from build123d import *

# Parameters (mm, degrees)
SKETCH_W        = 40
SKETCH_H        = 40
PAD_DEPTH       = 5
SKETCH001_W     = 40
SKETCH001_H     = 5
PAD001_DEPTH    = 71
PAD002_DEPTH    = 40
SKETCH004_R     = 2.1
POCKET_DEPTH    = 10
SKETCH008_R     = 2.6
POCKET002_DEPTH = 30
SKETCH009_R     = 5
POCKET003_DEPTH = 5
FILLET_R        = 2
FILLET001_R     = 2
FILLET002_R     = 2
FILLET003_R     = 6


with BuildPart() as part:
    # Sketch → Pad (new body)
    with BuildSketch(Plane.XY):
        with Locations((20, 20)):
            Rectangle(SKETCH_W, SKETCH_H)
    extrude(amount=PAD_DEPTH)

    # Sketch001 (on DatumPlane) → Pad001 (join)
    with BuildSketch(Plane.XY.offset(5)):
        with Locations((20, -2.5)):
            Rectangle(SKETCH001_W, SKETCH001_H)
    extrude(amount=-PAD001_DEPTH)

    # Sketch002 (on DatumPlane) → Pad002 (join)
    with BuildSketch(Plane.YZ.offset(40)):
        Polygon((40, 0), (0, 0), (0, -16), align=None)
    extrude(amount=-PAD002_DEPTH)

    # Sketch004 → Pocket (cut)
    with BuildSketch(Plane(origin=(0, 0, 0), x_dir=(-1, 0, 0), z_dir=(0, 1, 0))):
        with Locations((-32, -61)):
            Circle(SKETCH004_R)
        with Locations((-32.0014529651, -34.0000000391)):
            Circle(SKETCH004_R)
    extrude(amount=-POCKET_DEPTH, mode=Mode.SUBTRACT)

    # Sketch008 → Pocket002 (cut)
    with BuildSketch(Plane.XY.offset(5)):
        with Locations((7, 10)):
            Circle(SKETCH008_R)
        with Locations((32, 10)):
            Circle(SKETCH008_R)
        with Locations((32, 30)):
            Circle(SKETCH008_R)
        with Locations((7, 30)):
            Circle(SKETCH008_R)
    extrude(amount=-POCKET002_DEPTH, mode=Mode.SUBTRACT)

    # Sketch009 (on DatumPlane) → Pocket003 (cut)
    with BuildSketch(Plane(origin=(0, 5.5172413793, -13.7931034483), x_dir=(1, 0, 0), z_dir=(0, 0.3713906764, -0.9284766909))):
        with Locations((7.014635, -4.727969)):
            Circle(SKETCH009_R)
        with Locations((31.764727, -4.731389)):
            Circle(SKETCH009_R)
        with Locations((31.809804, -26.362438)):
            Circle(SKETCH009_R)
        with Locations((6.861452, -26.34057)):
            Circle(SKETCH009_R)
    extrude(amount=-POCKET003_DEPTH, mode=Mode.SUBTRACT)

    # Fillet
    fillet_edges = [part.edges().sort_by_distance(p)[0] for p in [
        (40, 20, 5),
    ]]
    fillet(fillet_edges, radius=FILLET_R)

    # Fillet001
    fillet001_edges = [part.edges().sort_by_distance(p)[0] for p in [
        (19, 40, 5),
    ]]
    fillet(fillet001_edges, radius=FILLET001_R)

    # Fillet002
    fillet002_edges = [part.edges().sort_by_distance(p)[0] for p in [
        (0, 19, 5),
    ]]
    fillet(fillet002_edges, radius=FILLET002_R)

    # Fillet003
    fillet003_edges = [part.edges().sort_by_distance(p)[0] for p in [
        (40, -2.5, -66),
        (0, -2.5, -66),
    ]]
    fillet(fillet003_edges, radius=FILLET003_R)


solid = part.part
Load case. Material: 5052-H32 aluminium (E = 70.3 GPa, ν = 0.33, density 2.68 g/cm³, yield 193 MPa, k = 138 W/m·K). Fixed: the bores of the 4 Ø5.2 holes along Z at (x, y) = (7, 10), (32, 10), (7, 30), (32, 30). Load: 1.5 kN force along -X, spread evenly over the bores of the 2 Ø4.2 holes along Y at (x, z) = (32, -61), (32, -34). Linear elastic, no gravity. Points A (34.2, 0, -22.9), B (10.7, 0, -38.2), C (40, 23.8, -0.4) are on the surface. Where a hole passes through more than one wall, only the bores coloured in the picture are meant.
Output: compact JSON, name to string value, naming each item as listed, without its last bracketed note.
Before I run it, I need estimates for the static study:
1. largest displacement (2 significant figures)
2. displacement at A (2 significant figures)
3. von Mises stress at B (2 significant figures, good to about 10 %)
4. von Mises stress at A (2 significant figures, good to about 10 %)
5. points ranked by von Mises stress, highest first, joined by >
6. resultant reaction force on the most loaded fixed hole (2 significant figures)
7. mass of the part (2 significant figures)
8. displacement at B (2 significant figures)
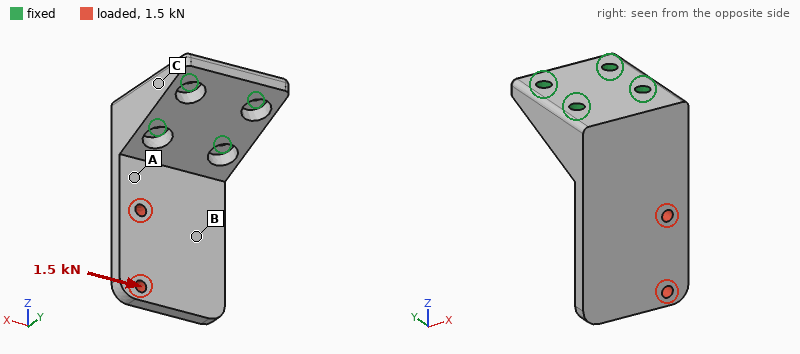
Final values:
{"largest displacement": "75 µm", "displacement at A": "21 µm", "von Mises stress at B": "13 MPa", "von Mises stress at A": "28 MPa", "points ranked by von Mises stress, highest first, joined by >": "A > B > C", "resultant reaction force on the most loaded fixed hole": "2.4 kN", "mass of the part": "87 g", "displacement at B": "36 µm"}
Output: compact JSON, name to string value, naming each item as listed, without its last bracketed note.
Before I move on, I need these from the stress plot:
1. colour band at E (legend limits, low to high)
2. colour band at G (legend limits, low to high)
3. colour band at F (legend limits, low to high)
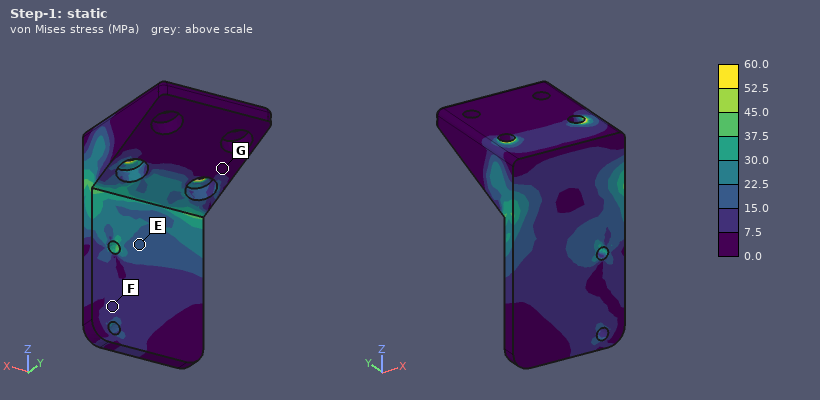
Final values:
{"colour band at E": "15.0 to 22.5 MPa", "colour band at G": "0.0 to 7.5 MPa", "colour band at F": "7.5 to 15.0 MPa"}
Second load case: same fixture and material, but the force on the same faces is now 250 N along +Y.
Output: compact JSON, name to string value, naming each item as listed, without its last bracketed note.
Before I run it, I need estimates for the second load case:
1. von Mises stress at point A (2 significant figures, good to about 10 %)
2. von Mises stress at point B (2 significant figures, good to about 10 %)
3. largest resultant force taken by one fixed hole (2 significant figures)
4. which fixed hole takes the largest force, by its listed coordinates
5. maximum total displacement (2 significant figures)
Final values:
{"von Mises stress at point A": "39 MPa", "von Mises stress at point B": "20 MPa", "largest resultant force taken by one fixed hole": "220 N", "which fixed hole takes the largest force, by its listed coordinates": "(32, 10)", "maximum total displacement": "0.26 mm"}
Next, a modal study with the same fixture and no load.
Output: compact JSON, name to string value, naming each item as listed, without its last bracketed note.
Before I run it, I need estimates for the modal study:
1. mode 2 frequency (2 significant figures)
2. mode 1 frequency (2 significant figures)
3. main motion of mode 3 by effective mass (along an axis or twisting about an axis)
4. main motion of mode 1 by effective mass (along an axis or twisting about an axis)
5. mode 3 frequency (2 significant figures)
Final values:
{"mode 2 frequency": "4300 Hz", "mode 1 frequency": "1500 Hz", "main motion of mode 3 by effective mass": "along X", "main motion of mode 1 by effective mass": "along Y", "mode 3 frequency": "6000 Hz"}
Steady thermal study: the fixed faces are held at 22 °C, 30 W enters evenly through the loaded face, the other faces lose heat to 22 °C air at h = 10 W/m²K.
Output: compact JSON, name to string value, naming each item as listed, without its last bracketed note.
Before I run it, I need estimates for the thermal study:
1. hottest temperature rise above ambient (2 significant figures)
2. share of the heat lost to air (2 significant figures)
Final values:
{"hottest temperature rise above ambient": "55 K", "share of the heat lost to air": "5.1 %"}
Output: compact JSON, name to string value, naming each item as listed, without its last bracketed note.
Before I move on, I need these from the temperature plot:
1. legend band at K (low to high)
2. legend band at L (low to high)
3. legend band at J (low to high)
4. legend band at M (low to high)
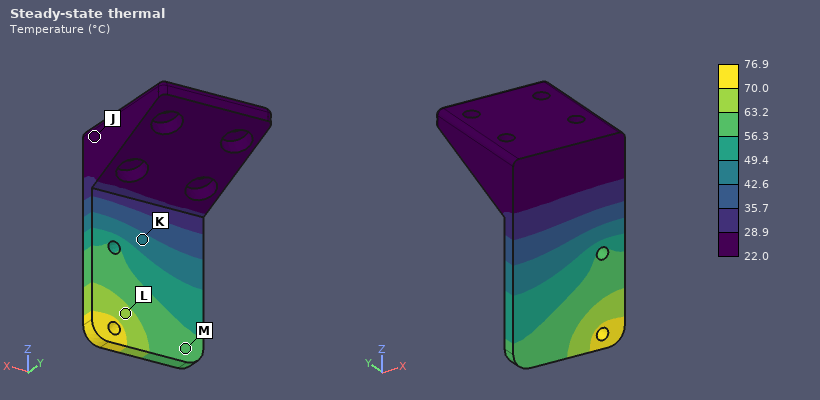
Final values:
{"legend band at K": "42.6 to 49.4 °C", "legend band at L": "63.2 to 70.0 °C", "legend band at J": "22.0 to 28.9 °C", "legend band at M": "56.3 to 63.2 °C"}
